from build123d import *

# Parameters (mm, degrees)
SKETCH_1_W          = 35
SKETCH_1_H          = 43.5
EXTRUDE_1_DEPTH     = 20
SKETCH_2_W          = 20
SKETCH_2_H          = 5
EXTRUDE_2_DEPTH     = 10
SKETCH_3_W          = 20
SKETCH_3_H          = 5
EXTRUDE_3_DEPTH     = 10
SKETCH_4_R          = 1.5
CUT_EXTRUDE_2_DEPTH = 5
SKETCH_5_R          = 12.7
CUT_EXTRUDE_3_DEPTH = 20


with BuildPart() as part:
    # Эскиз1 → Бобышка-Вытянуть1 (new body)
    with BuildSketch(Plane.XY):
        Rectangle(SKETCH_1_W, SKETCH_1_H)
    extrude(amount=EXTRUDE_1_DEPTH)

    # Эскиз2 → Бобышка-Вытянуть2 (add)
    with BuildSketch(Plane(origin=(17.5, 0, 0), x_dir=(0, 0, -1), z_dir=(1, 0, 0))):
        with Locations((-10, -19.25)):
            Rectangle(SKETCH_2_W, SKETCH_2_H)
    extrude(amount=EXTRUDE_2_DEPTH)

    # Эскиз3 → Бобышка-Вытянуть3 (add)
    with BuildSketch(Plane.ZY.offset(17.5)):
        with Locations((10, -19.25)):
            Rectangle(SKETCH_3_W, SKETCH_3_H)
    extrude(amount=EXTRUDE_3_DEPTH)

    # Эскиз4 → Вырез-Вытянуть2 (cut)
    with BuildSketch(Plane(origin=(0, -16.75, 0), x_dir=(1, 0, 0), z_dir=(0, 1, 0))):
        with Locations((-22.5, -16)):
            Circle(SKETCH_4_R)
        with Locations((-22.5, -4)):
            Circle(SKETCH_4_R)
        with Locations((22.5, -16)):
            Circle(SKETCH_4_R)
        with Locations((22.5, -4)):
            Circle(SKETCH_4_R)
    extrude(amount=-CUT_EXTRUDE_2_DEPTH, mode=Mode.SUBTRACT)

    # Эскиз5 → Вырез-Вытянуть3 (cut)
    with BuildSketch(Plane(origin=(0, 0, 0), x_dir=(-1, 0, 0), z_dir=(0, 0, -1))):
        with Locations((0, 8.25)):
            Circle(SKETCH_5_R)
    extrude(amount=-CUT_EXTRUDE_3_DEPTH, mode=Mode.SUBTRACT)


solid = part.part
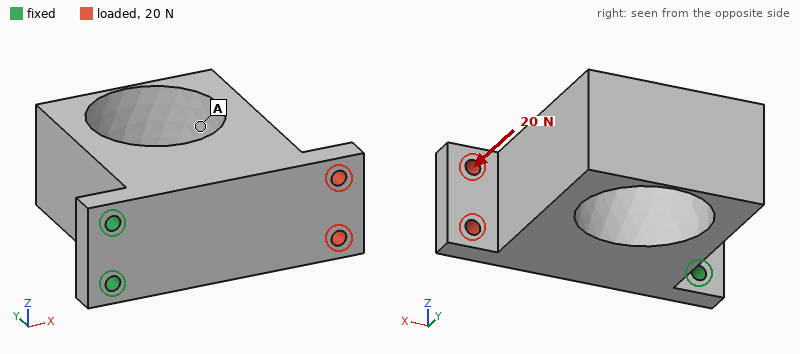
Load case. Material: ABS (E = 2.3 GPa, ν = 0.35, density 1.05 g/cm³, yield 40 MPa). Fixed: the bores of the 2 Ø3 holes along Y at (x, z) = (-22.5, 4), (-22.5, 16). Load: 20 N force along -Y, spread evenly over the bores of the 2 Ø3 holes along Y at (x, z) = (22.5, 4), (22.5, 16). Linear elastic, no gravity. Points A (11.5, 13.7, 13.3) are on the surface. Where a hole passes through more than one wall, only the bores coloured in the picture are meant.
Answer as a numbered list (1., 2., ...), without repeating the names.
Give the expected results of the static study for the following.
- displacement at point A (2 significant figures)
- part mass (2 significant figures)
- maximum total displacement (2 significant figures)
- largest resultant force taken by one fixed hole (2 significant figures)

1. 0.57 mm
2. 23 g
3. 0.70 mm
4. 10 N
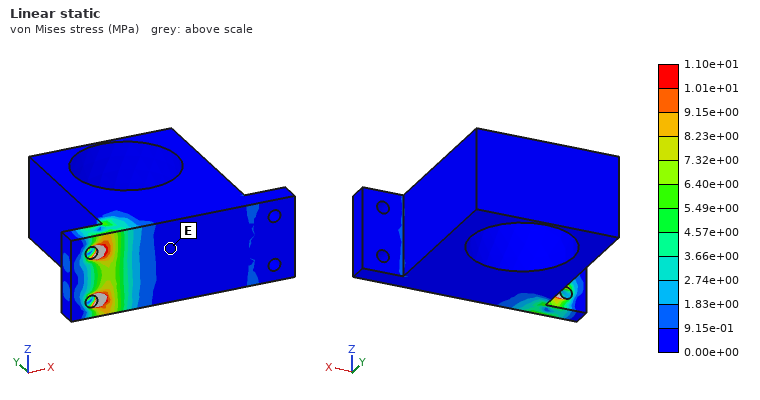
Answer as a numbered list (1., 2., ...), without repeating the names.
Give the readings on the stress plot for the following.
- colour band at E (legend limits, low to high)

1. 0.00e+00 to 9.15e-01 MPa
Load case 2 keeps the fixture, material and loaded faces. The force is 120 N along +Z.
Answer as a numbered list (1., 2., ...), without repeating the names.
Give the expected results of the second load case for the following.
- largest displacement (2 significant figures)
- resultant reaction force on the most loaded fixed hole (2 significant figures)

1. 0.49 mm
2. 400 N
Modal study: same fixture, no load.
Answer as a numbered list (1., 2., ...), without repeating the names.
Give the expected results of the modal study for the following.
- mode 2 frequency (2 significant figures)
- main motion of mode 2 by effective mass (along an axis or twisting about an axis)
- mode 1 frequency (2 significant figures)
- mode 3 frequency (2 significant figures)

1. 770 Hz
2. along Z
3. 280 Hz
4. 1300 Hz
